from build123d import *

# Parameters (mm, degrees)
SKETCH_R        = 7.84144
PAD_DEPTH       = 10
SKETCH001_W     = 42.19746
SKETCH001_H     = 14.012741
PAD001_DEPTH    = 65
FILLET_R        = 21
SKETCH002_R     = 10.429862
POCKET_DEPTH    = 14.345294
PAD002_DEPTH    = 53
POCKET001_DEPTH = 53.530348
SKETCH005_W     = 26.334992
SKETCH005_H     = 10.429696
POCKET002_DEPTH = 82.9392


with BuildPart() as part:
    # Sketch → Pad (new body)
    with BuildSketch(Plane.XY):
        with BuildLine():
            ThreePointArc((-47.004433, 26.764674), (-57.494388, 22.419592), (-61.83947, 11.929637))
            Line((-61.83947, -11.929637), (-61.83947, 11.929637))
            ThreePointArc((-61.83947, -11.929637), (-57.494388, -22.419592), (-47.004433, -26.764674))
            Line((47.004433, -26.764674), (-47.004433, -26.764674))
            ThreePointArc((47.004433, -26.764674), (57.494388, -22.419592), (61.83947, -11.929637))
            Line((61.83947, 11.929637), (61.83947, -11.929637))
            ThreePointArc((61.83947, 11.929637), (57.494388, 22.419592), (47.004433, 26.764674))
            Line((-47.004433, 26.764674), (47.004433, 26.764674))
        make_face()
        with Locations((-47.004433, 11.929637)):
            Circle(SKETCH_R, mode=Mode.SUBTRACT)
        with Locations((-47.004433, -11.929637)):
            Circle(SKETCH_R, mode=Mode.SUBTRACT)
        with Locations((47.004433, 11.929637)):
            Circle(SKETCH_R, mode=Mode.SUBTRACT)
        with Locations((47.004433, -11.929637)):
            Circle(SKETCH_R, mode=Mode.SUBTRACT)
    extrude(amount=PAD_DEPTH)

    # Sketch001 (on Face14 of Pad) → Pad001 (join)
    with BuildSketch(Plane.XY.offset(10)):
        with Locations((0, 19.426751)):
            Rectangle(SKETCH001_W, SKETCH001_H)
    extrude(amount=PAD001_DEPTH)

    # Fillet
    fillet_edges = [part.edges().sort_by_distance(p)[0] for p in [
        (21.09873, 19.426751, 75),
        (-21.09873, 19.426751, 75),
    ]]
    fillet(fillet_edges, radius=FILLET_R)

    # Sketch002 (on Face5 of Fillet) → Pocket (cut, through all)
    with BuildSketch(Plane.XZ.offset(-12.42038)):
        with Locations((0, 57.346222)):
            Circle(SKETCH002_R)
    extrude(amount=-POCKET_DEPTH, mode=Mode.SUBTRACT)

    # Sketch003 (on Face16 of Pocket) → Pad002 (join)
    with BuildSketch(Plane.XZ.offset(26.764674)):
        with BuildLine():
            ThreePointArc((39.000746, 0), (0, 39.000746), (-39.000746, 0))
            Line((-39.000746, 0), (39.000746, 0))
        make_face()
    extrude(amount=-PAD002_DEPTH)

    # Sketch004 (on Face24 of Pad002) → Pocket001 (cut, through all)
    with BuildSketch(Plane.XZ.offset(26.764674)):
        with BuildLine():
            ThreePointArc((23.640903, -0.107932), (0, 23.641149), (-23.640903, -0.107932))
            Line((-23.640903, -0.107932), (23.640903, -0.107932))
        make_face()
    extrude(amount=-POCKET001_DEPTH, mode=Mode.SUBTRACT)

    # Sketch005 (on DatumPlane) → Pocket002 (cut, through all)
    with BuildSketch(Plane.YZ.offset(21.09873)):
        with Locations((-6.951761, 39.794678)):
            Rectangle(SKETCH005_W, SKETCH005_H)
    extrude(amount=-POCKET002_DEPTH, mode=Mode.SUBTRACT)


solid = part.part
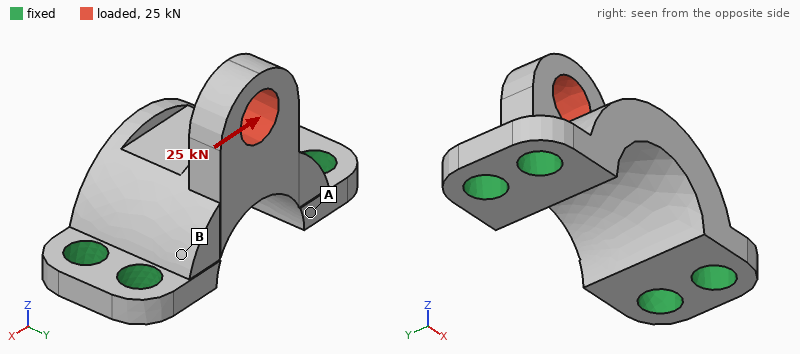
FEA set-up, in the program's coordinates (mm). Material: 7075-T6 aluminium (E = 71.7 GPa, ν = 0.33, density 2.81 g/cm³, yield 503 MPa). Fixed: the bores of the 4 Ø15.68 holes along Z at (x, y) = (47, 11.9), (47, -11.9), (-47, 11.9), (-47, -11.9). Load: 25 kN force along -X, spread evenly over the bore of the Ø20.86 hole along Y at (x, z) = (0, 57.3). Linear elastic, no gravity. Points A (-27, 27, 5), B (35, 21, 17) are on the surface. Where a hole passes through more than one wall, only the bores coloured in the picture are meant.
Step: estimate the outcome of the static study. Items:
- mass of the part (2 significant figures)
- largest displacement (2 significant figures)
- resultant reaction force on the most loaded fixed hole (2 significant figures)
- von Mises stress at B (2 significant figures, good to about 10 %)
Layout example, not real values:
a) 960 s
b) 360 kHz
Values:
a) 300 g
b) 0.30 mm
c) 14 kN
d) 80 MPa
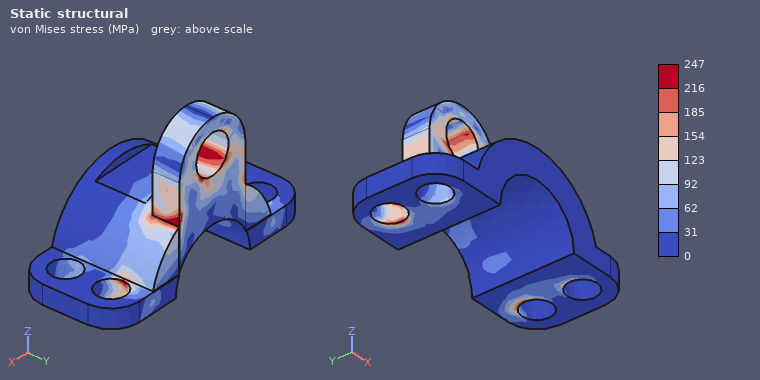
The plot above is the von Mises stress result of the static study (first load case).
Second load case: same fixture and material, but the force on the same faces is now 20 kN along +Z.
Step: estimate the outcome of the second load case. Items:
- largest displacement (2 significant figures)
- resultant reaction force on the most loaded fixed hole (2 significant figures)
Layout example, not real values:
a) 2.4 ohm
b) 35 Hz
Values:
a) 0.15 mm
b) 13 kN
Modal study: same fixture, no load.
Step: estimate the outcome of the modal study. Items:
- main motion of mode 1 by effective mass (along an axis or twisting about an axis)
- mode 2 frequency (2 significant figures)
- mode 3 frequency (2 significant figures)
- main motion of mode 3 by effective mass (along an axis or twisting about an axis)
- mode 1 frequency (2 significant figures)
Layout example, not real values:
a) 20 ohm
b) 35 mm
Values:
a) along Y
b) 8600 Hz
c) 9400 Hz
d) along Y
e) 4700 Hz
